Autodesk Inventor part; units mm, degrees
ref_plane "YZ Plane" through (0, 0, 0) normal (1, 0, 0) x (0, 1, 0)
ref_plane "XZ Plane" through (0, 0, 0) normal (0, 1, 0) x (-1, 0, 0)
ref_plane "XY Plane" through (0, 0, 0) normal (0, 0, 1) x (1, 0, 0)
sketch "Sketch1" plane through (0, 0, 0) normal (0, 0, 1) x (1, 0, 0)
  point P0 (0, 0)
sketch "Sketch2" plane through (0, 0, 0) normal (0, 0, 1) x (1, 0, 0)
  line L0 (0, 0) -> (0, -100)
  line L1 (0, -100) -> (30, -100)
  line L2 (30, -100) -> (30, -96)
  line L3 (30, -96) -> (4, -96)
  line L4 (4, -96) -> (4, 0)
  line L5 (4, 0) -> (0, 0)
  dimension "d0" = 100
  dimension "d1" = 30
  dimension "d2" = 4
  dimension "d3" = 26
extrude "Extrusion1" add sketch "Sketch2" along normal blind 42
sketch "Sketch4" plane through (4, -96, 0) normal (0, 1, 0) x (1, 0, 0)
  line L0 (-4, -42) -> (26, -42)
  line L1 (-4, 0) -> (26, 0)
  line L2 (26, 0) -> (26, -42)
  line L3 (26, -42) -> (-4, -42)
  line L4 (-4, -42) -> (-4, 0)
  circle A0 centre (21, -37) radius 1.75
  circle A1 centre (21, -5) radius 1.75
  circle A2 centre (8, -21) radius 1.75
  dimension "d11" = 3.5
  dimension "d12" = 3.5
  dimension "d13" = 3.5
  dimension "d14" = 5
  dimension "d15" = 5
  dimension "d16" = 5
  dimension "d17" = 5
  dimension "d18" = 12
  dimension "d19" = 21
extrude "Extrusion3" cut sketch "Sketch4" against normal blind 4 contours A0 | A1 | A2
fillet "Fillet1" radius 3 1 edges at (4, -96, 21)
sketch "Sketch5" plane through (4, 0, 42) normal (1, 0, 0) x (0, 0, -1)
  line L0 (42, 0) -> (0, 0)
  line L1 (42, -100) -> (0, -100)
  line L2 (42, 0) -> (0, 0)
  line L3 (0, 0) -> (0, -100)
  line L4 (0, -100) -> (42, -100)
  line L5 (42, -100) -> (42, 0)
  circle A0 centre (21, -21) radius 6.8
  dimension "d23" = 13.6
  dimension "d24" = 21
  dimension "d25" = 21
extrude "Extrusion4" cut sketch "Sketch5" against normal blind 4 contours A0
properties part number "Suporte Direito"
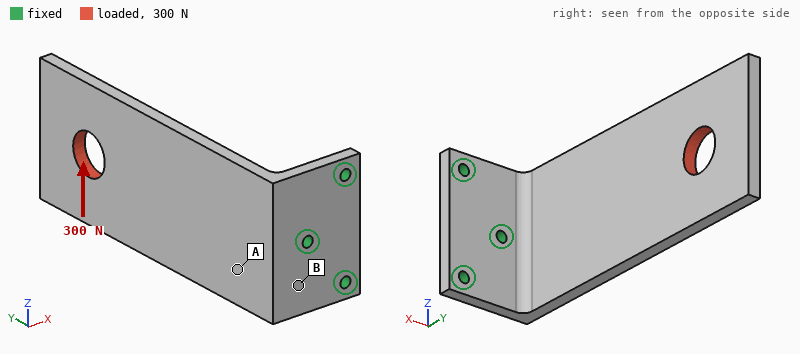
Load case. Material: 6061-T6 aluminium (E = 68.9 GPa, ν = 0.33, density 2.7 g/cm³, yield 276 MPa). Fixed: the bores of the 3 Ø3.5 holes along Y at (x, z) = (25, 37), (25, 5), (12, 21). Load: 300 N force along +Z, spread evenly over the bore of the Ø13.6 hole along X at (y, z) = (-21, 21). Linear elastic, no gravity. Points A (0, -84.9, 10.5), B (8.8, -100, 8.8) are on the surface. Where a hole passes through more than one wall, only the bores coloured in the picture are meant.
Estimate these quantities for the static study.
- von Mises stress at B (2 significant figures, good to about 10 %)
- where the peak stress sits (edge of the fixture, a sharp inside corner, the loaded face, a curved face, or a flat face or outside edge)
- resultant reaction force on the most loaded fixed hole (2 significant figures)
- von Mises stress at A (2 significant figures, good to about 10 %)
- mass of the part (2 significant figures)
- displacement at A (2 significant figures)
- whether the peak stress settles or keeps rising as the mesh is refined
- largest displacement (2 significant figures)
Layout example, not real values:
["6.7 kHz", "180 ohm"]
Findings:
["60 MPa", "edge of the fixture", "420 N", "21 MPa", "55 g", "0.12 mm", "keeps rising", "0.77 mm"]
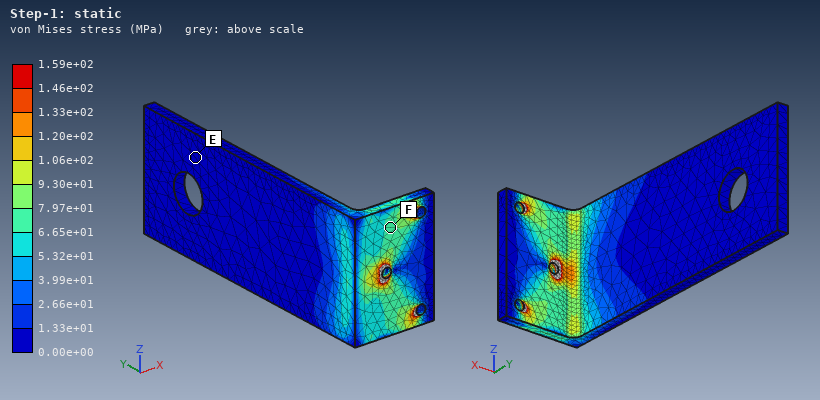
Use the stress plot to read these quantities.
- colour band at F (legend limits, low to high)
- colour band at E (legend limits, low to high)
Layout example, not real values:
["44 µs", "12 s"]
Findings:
["6.65e+01 to 7.97e+01 MPa", "0.00e+00 to 1.33e+01 MPa"]
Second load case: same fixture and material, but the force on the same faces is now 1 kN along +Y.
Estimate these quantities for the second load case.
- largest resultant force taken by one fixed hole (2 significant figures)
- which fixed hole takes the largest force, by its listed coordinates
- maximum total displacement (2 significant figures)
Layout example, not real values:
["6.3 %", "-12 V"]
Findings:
["1.2 kN", "(12, 21)", "0.43 mm"]
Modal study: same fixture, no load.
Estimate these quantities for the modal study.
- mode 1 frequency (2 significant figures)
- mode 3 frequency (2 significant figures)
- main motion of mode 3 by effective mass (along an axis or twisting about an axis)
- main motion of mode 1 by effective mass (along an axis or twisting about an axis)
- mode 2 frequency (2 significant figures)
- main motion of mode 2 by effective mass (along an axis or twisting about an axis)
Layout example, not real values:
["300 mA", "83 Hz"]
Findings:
["310 Hz", "1600 Hz", "twisting about Y", "along X", "740 Hz", "along Z"]
